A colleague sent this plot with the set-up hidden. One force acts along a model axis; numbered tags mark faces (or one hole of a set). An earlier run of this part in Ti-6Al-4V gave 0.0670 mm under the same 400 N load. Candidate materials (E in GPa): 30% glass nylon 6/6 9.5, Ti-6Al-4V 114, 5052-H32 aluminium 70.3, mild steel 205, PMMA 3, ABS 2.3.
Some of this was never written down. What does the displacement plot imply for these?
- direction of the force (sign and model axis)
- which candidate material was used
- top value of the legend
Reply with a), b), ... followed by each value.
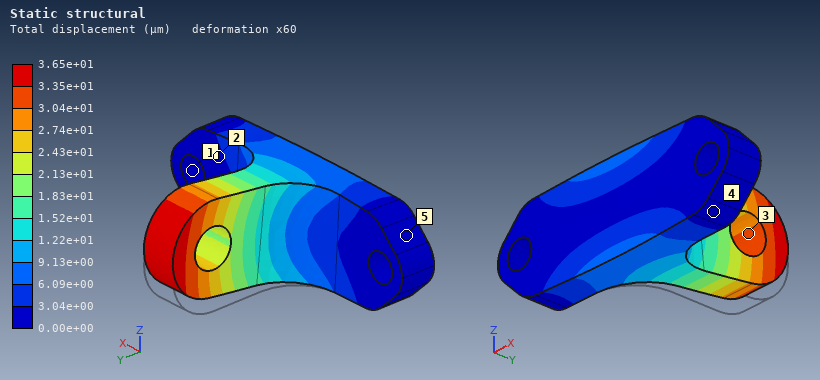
a) +Z
b) mild steel
c) 3.65e+01 µm
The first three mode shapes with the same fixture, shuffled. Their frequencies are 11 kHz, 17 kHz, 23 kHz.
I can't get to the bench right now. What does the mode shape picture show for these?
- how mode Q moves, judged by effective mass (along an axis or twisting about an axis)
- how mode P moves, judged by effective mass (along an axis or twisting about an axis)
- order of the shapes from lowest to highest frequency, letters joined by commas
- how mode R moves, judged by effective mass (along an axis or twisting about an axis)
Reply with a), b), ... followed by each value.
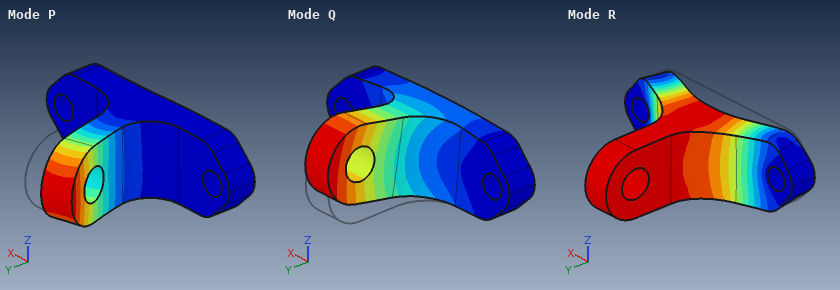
a) along Z
b) along X
c) Q, P, R
d) along Y
